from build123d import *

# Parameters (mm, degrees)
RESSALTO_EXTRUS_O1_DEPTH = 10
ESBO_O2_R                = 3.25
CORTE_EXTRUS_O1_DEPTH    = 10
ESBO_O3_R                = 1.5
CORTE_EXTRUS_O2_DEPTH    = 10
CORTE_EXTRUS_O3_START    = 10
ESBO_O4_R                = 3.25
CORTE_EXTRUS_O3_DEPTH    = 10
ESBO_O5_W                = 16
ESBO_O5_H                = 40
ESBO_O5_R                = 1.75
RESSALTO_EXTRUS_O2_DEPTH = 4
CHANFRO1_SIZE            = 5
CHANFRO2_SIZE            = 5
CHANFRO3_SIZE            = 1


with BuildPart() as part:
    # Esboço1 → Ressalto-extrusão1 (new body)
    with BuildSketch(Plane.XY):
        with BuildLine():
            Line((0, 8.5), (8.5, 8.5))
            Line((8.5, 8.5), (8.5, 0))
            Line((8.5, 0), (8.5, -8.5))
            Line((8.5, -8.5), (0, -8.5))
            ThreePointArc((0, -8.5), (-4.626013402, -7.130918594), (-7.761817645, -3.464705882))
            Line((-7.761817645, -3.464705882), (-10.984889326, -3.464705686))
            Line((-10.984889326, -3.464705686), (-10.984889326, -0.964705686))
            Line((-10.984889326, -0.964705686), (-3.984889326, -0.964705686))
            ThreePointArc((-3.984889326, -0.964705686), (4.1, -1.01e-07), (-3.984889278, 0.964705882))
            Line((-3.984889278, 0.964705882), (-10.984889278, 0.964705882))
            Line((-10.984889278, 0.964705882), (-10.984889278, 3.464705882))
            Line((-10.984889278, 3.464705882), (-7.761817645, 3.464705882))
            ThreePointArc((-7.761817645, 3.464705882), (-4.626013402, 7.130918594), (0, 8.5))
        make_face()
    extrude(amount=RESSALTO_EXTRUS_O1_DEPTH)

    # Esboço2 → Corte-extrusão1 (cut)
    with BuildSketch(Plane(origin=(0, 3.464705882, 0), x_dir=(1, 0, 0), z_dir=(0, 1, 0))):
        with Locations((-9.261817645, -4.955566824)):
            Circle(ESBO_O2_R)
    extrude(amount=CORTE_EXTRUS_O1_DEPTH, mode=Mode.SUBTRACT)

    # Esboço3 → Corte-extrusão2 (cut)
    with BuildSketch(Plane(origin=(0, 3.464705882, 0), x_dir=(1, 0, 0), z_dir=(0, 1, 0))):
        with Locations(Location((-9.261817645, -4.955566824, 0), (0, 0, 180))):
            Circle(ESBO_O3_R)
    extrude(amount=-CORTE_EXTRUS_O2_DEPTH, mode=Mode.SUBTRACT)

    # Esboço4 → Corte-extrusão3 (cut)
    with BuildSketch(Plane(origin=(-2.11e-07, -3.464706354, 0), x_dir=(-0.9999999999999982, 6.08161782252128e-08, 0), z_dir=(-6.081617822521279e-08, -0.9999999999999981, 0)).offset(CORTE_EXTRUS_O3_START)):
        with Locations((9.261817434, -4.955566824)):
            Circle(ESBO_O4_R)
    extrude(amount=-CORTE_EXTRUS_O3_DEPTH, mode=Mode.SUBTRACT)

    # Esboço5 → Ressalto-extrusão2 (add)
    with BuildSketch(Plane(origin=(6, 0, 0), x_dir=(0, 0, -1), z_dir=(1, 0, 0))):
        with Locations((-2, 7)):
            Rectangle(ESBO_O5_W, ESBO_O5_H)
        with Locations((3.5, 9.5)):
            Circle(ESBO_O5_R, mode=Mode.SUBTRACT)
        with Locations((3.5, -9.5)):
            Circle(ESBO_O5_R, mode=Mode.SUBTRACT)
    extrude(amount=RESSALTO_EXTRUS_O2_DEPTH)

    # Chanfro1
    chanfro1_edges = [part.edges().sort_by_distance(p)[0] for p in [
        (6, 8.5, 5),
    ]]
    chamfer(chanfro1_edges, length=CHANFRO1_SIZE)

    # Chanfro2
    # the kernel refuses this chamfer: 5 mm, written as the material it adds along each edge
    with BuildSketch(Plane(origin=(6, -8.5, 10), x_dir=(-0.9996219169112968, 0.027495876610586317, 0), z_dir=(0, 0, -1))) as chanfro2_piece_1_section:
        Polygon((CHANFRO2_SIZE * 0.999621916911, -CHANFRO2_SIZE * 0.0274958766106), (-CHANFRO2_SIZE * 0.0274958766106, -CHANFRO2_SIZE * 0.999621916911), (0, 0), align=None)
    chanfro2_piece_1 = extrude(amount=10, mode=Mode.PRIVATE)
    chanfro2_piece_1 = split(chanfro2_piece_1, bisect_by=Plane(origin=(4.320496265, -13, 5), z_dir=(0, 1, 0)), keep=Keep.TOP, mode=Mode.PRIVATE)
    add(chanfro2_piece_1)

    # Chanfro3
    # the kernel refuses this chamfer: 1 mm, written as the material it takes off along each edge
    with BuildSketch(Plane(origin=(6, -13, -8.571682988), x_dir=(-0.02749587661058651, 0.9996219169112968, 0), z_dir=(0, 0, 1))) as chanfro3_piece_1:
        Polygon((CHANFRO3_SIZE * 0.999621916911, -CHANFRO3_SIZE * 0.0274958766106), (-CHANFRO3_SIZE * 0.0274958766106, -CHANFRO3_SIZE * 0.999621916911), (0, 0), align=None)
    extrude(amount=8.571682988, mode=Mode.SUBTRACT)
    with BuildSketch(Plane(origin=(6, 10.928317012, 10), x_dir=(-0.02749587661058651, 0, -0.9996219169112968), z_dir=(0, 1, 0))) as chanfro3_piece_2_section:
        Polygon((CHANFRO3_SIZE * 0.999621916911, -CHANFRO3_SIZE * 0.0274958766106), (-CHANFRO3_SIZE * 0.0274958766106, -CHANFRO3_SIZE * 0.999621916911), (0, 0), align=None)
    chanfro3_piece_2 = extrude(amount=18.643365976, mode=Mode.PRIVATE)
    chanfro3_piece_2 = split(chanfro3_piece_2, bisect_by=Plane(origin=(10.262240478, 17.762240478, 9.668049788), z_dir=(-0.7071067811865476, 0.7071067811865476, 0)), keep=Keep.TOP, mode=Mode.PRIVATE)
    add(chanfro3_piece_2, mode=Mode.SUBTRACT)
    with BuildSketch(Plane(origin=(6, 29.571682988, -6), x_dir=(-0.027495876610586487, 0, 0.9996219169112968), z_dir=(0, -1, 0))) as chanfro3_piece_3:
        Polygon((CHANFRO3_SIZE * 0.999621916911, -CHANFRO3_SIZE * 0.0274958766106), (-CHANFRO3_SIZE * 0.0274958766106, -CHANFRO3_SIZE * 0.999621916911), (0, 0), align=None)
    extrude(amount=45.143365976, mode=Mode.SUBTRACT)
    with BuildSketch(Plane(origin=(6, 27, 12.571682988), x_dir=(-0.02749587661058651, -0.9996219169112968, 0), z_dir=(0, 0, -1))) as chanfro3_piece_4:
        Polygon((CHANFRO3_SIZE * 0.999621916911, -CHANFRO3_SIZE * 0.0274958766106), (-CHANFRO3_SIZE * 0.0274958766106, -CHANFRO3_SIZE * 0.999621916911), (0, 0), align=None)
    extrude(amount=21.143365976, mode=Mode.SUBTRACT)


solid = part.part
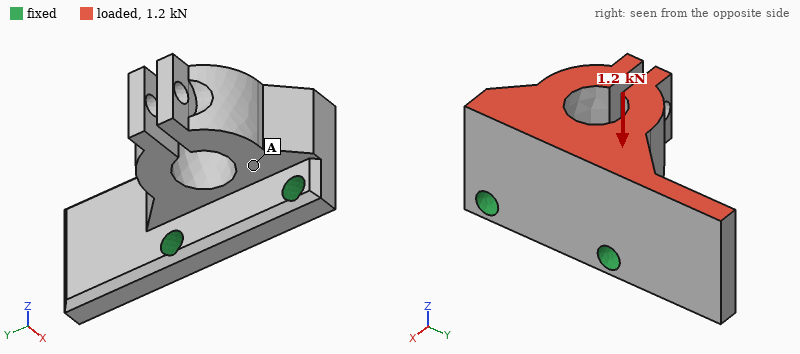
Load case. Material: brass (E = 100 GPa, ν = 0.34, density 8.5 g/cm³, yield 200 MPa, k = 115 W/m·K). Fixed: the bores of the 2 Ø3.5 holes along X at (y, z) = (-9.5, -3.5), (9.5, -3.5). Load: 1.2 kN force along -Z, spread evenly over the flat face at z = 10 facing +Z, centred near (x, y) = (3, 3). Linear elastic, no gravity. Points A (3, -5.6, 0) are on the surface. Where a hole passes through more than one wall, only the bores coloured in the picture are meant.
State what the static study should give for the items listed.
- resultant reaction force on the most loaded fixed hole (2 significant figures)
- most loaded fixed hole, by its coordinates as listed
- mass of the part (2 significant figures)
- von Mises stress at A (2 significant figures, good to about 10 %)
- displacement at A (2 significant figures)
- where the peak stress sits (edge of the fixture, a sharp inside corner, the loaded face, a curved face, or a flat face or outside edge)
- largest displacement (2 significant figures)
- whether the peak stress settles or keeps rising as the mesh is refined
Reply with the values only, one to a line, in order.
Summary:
740 N
(9.5, -3.5)
37 g
20 MPa
12 µm
edge of the fixture
54 µm
keeps rising
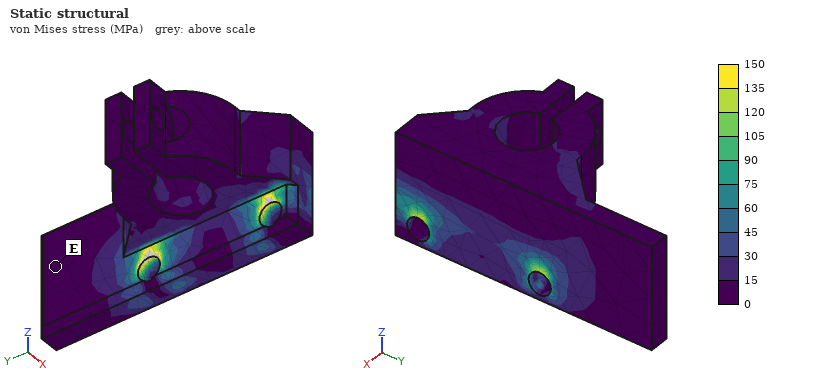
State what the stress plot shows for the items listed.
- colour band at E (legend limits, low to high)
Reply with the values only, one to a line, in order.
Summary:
0 to 15 MPa
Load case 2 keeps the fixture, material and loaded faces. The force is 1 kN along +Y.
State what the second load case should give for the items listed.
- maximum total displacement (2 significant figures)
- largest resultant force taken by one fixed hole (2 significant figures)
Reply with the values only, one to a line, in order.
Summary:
20 µm
830 N
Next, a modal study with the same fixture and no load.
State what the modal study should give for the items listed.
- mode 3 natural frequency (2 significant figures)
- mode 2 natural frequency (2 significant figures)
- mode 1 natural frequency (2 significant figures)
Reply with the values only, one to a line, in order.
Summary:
9900 Hz
6900 Hz
4800 Hz
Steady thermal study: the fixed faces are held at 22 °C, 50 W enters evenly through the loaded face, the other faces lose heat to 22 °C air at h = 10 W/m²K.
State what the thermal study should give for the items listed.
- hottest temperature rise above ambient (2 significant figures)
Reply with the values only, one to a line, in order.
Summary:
48 K
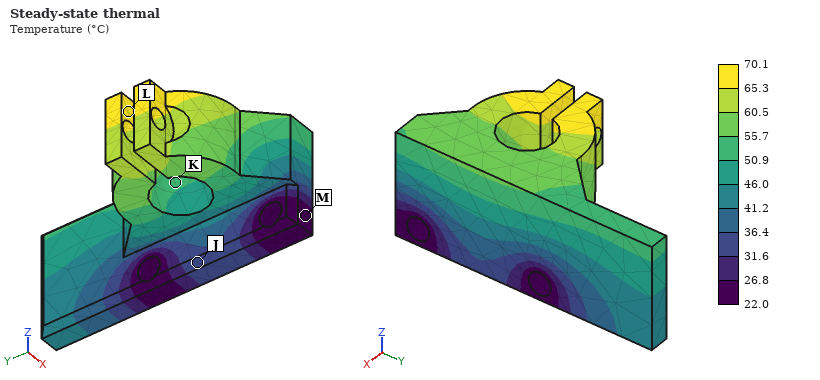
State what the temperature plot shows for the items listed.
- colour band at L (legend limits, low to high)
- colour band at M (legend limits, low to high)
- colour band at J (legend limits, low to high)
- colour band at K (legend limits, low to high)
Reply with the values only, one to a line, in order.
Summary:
65.3 to 70.1 °C
22.0 to 26.8 °C
31.6 to 36.4 °C
50.9 to 55.7 °C
